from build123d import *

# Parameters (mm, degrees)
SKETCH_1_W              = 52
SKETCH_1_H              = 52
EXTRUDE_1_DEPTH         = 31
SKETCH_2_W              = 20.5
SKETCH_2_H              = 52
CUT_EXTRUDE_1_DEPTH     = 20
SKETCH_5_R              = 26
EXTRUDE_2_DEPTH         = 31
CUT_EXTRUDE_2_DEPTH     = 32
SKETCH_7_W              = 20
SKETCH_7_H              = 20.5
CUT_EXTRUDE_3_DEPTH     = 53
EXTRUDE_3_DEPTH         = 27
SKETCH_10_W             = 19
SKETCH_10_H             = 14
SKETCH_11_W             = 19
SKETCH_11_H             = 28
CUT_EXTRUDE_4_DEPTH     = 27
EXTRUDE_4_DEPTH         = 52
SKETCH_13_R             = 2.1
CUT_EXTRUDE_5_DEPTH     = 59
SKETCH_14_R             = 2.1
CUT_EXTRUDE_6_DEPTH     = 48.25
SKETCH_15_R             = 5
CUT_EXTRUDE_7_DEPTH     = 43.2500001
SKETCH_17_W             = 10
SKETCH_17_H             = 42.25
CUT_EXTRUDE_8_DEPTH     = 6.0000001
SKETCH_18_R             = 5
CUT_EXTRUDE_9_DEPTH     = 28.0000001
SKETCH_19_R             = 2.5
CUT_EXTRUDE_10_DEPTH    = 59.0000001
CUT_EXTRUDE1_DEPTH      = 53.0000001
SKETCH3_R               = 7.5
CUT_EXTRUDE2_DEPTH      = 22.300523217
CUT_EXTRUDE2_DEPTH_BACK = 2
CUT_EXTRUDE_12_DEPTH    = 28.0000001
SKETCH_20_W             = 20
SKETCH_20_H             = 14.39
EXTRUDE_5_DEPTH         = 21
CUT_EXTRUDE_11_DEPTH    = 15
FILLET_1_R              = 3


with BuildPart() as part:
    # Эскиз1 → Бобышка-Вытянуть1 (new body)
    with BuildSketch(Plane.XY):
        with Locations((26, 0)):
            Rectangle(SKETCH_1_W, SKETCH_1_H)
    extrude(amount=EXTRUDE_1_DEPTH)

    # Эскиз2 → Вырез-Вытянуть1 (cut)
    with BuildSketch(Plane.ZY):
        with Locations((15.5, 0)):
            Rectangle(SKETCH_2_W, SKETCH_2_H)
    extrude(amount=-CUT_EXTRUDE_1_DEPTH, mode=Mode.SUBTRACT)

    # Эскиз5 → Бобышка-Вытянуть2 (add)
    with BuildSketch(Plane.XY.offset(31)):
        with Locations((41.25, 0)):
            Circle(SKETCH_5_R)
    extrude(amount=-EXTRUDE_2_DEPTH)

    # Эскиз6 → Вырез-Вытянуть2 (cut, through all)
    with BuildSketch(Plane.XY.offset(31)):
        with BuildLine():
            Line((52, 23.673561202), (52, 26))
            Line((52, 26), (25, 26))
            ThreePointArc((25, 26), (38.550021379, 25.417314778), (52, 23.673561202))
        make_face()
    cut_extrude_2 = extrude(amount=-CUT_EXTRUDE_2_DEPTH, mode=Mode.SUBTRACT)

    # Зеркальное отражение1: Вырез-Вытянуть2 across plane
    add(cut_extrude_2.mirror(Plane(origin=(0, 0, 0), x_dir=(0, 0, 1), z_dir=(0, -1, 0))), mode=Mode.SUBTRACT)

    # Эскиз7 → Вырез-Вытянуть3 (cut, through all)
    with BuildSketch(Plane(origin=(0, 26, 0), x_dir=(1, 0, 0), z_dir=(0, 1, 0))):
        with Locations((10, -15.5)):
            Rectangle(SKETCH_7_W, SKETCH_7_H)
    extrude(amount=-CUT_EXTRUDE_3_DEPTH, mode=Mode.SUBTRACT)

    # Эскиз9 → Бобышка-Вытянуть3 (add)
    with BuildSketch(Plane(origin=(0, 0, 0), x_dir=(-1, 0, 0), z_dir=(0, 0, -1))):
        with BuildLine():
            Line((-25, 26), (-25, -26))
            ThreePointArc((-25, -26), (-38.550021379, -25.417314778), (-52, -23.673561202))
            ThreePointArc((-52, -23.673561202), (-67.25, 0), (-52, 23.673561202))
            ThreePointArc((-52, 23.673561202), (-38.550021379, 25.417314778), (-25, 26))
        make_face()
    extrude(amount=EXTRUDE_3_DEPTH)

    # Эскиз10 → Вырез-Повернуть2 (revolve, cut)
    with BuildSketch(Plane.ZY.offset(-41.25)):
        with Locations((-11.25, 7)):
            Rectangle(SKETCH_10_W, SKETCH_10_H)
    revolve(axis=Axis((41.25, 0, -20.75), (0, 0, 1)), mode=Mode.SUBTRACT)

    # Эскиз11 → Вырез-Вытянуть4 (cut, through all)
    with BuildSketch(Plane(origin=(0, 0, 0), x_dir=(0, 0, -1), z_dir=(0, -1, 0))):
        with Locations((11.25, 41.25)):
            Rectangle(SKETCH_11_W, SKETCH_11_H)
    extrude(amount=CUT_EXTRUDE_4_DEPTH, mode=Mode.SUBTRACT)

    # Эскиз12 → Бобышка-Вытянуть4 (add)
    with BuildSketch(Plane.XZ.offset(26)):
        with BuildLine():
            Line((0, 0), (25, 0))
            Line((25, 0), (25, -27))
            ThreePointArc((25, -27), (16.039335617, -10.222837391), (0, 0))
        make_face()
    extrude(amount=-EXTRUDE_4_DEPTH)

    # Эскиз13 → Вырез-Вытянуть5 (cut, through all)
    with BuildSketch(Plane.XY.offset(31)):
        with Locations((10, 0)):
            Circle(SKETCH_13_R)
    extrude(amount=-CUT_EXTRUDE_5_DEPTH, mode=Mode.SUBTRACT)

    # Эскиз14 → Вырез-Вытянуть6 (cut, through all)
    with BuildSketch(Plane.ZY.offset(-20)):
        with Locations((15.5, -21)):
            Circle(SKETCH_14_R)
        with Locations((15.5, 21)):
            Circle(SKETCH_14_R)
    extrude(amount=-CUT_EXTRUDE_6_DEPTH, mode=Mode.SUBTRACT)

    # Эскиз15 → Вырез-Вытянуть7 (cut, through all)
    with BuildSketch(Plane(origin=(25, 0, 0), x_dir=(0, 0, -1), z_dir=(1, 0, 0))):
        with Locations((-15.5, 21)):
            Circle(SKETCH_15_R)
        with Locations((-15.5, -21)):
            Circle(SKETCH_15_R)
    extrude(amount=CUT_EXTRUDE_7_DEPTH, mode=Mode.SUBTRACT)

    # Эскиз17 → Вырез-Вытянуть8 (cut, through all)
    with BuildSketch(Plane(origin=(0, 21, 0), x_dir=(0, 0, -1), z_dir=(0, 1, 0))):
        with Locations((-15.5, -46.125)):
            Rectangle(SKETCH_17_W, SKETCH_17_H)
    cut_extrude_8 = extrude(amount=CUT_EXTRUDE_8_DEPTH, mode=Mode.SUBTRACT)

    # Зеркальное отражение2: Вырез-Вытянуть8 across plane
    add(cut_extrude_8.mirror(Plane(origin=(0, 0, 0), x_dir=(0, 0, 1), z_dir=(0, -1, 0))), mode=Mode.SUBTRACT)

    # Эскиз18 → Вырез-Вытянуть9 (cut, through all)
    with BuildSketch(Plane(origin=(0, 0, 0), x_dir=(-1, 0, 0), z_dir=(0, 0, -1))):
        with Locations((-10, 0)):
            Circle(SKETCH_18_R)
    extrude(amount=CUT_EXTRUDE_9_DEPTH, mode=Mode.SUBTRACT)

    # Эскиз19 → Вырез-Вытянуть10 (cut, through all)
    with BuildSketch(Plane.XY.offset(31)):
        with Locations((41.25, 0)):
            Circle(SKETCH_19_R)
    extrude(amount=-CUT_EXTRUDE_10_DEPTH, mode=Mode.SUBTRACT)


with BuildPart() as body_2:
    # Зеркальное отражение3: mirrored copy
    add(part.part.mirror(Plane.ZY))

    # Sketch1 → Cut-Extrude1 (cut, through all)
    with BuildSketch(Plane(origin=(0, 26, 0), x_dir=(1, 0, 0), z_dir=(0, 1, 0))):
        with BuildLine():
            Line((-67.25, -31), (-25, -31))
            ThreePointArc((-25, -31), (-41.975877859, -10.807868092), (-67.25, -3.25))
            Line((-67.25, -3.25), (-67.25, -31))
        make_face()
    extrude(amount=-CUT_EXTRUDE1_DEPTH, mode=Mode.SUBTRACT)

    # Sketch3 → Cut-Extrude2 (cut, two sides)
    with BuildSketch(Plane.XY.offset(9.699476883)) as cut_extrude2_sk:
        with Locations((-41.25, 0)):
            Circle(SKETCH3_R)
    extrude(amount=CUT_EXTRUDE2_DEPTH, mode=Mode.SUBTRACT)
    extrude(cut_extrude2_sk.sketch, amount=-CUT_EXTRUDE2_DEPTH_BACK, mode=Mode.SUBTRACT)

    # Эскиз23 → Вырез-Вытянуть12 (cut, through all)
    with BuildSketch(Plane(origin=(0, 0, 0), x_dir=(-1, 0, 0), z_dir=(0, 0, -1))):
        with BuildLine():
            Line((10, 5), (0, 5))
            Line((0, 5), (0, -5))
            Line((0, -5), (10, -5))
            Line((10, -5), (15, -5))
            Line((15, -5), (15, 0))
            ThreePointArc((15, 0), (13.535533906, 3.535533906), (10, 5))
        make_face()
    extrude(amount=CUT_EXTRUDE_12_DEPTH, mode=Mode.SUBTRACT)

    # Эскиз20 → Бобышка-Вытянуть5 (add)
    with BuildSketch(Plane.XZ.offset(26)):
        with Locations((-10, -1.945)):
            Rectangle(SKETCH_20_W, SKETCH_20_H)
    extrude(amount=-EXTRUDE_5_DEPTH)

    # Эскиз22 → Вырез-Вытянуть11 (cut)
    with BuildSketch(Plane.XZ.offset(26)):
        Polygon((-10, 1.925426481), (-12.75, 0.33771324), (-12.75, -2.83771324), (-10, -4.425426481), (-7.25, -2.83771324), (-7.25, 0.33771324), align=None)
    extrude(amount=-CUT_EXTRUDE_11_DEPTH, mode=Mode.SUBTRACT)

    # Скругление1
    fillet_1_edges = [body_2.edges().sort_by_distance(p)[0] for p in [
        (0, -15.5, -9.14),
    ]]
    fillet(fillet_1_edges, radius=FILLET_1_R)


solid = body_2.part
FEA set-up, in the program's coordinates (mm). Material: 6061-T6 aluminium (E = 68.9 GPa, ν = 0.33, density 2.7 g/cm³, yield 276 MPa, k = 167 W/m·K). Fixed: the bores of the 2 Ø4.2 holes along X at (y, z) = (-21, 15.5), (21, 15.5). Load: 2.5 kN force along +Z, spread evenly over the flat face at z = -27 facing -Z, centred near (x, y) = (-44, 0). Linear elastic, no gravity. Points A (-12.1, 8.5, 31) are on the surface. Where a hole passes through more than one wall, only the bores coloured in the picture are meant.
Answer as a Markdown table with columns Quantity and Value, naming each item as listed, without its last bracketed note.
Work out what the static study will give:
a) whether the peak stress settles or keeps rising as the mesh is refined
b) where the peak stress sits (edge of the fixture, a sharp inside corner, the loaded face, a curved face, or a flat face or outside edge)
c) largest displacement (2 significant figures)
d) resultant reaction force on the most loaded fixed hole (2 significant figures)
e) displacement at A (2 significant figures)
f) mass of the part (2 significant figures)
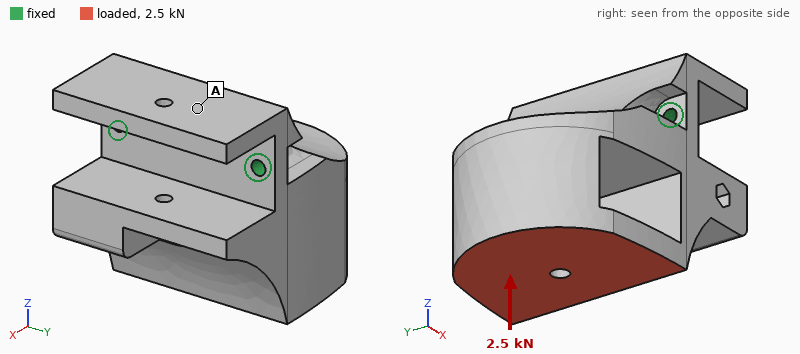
| Quantity | Value |
|---|---|
| whether the peak stress settles or keeps rising as the mesh is refined | keeps rising |
| where the peak stress sits | edge of the fixture |
| largest displacement | 0.34 mm |
| resultant reaction force on the most loaded fixed hole | 1.3 kN |
| displacement at A | 0.091 mm |
| mass of the part | 220 g |
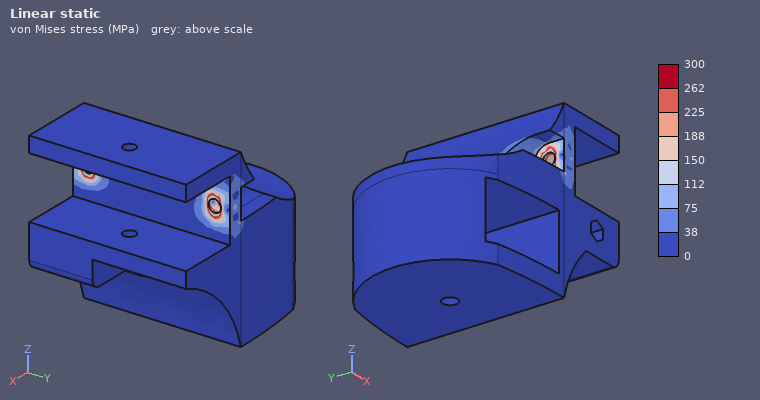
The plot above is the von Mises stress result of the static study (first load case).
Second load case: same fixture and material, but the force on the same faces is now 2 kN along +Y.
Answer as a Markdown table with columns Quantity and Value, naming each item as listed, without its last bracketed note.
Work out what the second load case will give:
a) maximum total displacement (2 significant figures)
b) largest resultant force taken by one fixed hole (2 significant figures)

| Quantity | Value |
|---|---|
| maximum total displacement | 31 µm |
| largest resultant force taken by one fixed hole | 2.5 kN |
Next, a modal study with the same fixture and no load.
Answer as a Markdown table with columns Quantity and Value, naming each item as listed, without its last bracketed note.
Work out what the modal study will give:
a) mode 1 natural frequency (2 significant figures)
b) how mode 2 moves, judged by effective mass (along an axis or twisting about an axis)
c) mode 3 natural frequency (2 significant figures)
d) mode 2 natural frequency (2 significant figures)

| Quantity | Value |
|---|---|
| mode 1 natural frequency | 1100 Hz |
| how mode 2 moves, judged by effective mass | along Y |
| mode 3 natural frequency | 6400 Hz |
| mode 2 natural frequency | 5000 Hz |
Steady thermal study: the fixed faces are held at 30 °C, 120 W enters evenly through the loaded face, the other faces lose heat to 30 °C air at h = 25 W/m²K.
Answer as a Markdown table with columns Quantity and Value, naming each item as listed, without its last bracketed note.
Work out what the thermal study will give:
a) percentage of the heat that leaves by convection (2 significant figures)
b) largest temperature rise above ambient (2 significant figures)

| Quantity | Value |
|---|---|
| percentage of the heat that leaves by convection | 12 % |
| largest temperature rise above ambient | 58 K |
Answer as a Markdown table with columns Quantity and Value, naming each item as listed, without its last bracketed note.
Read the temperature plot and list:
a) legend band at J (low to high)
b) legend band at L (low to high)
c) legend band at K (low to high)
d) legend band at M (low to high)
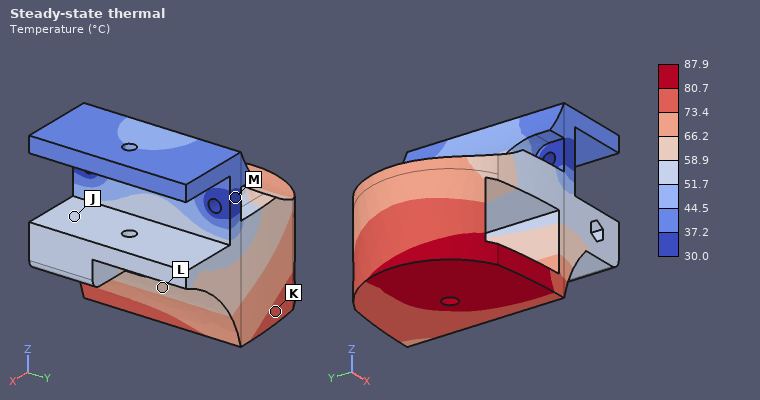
| Quantity | Value |
|---|---|
| legend band at J | 51.7 to 58.9 °C |
| legend band at L | 58.9 to 66.2 °C |
| legend band at K | 73.4 to 80.7 °C |
| legend band at M | 30.0 to 37.2 °C |
